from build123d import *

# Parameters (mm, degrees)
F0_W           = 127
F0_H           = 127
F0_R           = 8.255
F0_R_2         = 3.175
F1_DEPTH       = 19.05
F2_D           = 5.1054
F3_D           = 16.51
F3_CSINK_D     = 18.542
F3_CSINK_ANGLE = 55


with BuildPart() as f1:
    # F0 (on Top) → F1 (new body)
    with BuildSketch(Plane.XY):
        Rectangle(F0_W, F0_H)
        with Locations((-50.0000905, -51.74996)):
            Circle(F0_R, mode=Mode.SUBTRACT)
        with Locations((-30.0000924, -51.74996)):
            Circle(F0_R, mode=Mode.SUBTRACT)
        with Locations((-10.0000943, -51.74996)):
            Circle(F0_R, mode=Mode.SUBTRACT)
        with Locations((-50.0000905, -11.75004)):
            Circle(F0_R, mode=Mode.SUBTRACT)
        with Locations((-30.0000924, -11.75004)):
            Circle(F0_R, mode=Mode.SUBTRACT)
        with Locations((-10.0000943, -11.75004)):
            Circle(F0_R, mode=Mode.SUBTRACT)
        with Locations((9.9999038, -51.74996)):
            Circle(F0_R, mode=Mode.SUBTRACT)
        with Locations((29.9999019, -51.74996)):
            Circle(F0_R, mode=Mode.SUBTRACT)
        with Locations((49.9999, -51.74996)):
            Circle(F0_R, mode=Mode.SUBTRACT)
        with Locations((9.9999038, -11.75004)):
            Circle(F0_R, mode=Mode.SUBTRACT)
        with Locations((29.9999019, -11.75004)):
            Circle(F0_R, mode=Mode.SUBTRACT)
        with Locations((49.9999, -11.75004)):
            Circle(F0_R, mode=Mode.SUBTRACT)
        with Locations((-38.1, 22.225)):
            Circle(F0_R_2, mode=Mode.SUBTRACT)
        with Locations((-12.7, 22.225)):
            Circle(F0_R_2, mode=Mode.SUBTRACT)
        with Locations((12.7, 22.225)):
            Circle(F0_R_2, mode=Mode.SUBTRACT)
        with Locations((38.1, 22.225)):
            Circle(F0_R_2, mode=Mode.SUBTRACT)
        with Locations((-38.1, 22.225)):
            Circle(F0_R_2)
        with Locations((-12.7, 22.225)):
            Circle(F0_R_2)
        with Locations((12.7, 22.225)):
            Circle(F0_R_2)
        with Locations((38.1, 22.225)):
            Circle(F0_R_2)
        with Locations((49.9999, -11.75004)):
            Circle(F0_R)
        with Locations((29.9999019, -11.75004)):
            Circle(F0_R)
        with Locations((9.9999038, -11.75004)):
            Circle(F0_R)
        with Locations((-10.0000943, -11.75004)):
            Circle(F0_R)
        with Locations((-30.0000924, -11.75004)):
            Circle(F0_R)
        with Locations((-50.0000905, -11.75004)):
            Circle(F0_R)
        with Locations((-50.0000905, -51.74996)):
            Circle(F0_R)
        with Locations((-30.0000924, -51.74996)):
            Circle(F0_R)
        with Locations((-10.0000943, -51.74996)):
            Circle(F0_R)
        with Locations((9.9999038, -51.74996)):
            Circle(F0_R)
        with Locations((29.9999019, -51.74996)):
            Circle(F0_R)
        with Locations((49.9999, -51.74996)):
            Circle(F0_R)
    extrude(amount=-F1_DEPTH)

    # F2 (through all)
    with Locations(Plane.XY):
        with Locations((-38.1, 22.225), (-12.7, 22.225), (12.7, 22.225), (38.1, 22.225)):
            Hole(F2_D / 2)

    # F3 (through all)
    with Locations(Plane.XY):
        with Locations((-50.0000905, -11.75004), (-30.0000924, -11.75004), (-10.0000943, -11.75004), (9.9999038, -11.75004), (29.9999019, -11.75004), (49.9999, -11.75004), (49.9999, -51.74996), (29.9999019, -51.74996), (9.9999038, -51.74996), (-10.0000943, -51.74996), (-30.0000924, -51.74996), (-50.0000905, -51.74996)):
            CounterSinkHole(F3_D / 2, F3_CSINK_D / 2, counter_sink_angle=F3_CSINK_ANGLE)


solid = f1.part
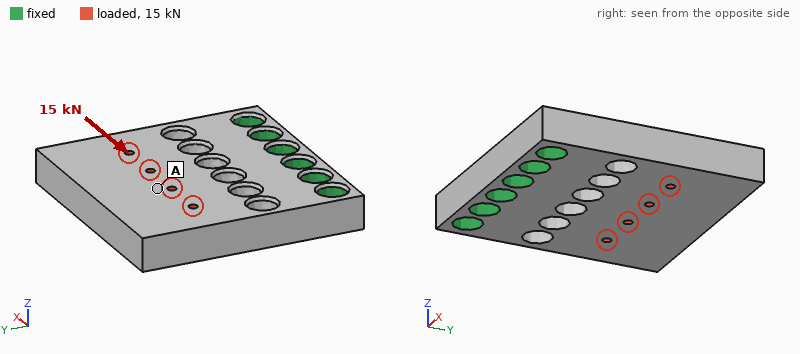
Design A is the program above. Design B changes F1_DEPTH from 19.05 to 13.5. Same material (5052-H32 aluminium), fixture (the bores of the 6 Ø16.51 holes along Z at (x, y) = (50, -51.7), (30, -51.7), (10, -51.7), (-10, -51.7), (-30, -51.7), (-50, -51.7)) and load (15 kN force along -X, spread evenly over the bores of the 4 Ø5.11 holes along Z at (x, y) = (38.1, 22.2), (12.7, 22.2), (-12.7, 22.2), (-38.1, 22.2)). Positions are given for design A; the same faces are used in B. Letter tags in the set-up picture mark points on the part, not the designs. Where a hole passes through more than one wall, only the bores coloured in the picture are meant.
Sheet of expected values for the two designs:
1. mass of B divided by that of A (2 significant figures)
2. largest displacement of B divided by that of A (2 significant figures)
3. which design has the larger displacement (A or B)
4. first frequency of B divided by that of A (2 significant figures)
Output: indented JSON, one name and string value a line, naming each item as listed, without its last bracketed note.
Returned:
{
  "mass of B divided by that of A": "0.71",
  "largest displacement of B divided by that of A": "1.5",
  "which design has the larger displacement": "B",
  "first frequency of B divided by that of A": "0.72"
}
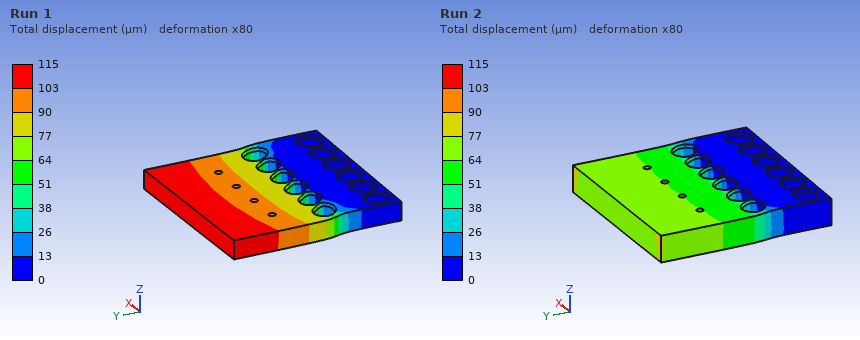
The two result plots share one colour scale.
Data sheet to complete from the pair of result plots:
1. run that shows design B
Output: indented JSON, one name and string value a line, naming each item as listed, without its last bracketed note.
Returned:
{
  "run that shows design B": "Run 1"
}
